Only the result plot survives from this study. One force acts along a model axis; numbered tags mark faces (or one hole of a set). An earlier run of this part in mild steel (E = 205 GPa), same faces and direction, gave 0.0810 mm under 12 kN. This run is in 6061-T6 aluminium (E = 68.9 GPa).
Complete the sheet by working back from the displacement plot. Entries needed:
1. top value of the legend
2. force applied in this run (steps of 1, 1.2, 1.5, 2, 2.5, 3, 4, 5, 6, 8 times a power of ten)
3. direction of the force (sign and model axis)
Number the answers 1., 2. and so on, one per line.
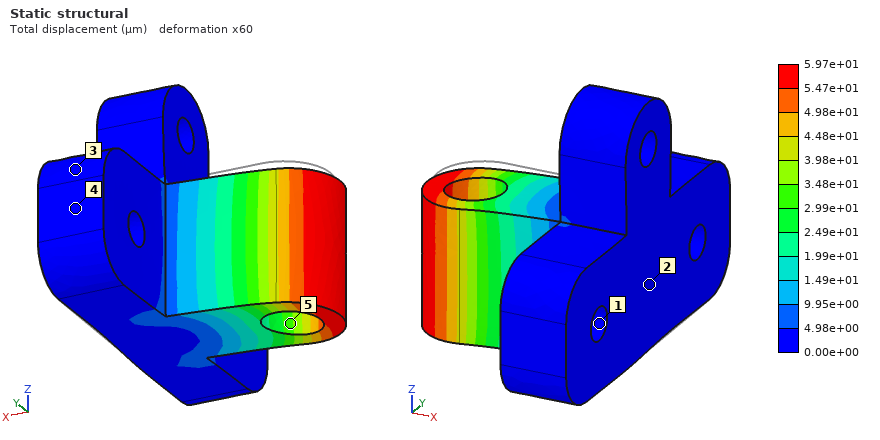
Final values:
1. 5.97e+01 µm
2. 3 kN
3. -Y
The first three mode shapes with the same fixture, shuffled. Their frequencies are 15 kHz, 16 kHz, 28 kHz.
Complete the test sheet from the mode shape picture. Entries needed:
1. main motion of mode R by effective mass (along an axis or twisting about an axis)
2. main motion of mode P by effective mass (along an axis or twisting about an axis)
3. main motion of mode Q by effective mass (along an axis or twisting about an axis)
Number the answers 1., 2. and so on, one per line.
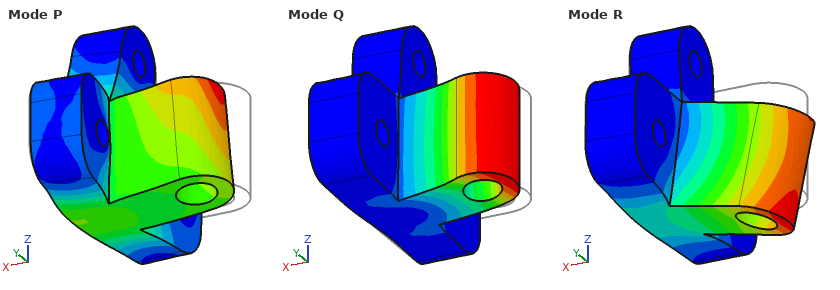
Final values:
1. along Z
2. along X
3. along Y
